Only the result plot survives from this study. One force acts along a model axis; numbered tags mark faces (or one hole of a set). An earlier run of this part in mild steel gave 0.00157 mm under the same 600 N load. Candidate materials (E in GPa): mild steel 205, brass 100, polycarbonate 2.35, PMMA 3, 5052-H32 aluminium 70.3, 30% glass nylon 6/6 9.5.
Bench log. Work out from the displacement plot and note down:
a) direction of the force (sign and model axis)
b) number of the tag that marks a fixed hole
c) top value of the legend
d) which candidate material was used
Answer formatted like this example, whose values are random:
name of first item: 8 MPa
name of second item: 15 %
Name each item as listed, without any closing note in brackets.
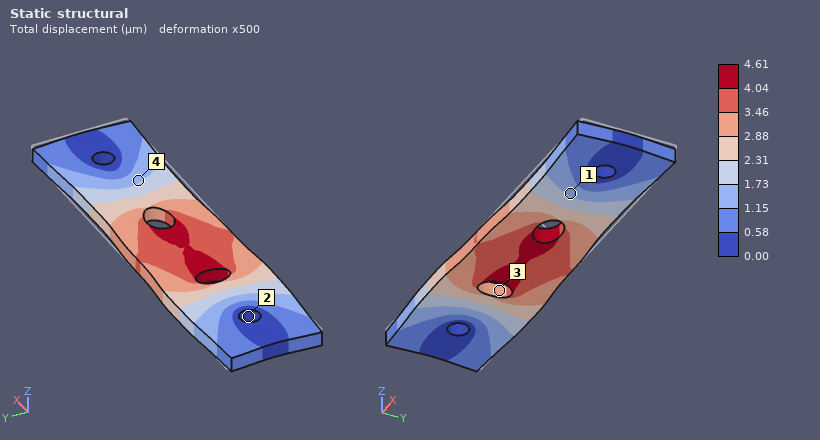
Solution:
direction of the force: -X
number of the tag that marks a fixed hole: 2
top value of the legend: 4.61 µm
which candidate material was used: 5052-H32 aluminium
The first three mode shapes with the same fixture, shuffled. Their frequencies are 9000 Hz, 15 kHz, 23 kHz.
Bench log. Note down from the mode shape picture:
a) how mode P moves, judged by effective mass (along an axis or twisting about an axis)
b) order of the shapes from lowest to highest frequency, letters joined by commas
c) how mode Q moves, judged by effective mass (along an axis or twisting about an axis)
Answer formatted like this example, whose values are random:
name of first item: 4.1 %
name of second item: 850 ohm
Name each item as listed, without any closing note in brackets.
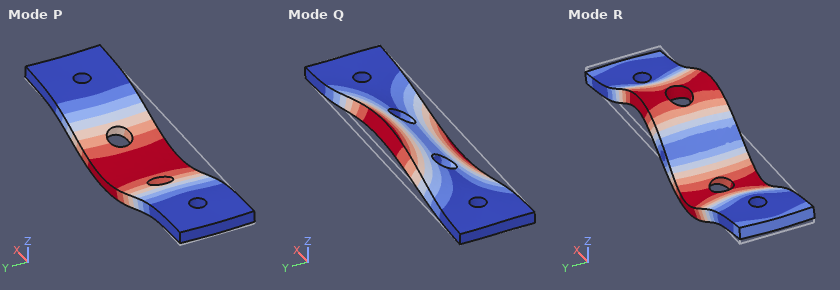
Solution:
how mode P moves, judged by effective mass: along Z
order of the shapes from lowest to highest frequency, letters joined by commas: P, Q, R
how mode Q moves, judged by effective mass: twisting about X
